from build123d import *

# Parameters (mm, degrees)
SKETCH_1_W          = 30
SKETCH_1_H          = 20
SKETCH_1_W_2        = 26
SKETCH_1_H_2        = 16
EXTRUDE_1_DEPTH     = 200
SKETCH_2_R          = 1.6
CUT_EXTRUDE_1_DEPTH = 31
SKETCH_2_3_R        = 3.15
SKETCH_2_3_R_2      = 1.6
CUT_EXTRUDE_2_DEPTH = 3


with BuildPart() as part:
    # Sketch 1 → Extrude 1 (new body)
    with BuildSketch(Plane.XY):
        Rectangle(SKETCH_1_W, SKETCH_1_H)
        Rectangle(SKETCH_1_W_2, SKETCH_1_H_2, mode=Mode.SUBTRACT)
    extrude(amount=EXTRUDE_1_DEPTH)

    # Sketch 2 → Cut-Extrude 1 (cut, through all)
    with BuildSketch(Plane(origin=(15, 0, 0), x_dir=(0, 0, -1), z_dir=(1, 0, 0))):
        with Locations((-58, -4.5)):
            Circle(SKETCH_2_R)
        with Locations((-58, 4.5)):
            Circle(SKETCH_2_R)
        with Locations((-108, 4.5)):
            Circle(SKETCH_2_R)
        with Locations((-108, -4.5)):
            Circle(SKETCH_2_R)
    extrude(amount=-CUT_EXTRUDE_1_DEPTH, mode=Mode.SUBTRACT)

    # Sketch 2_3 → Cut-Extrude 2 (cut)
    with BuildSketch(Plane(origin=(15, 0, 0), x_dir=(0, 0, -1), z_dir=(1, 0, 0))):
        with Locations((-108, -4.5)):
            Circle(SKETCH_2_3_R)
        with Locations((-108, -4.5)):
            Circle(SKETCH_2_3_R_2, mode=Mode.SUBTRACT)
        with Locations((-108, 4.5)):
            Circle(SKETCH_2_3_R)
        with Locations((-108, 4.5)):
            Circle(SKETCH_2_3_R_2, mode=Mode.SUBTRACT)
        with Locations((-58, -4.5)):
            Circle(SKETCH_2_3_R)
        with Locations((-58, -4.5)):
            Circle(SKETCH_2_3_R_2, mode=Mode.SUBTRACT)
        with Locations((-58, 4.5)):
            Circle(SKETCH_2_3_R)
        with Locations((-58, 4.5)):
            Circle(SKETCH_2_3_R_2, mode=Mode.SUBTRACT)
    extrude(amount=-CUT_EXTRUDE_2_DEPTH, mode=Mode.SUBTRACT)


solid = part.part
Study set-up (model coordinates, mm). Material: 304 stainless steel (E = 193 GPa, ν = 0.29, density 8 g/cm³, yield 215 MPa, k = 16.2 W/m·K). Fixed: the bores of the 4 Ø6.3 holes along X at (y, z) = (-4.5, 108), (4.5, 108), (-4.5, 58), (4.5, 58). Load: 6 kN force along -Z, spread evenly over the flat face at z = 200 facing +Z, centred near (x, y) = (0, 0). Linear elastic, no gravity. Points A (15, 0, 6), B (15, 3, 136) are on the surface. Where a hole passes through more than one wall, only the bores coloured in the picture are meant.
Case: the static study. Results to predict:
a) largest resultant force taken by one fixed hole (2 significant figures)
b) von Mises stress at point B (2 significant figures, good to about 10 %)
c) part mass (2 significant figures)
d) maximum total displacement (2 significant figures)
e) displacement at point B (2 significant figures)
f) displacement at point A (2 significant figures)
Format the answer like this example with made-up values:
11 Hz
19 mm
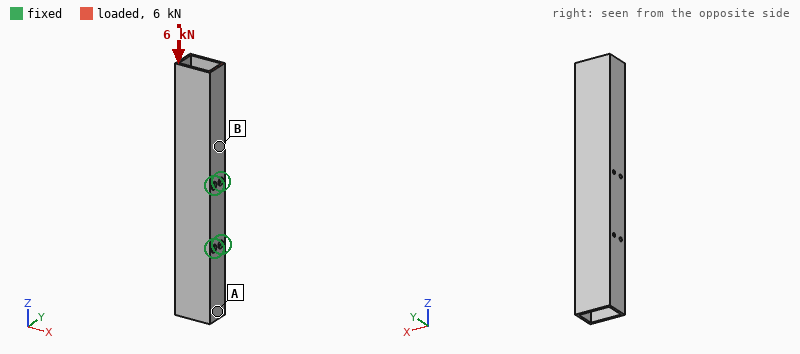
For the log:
2.2 kN
36 MPa
290 g
58 µm
17 µm
18 µm
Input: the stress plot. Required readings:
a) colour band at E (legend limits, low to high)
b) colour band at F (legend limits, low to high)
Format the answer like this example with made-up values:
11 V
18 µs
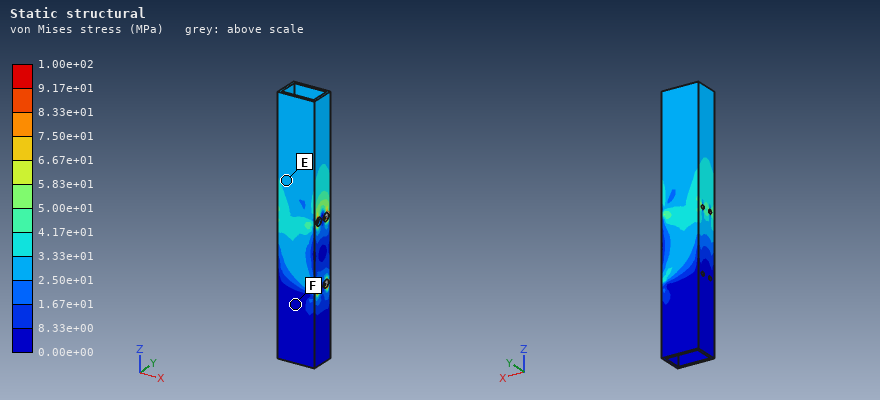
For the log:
2.50e+01 to 3.33e+01 MPa
0.00e+00 to 8.33e+00 MPa
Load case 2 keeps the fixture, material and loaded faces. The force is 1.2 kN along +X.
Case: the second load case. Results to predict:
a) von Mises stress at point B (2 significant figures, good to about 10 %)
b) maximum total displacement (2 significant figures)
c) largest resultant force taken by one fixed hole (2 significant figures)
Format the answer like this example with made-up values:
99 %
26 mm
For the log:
51 MPa
0.17 mm
2.0 kN
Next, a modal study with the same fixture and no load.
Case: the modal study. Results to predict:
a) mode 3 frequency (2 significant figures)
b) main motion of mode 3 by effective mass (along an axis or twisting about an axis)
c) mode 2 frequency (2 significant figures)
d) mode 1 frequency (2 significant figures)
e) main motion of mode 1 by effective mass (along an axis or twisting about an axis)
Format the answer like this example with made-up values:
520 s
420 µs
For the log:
2100 Hz
along X
1900 Hz
1400 Hz
along Y
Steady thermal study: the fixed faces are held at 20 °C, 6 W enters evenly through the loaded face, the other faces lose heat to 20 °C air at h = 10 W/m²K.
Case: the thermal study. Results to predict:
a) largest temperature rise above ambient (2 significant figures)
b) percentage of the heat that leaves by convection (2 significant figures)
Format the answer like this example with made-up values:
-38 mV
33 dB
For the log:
80 K
86 %
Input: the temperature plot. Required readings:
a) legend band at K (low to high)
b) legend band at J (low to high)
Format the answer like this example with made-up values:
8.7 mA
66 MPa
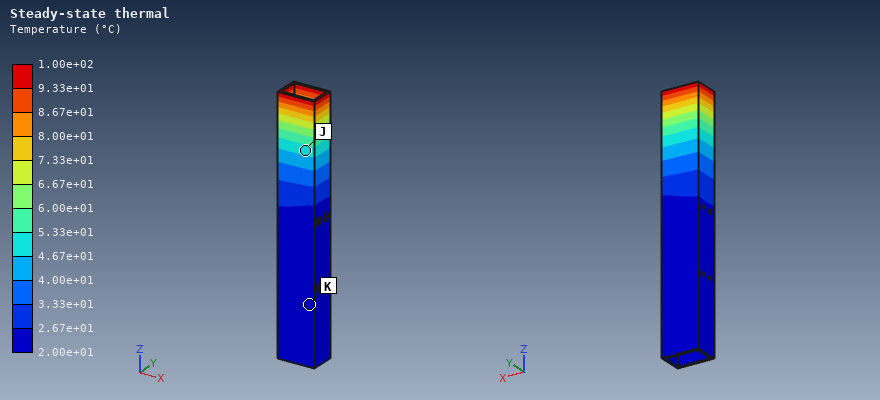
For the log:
2.00e+01 to 2.67e+01 °C
4.67e+01 to 5.33e+01 °C
